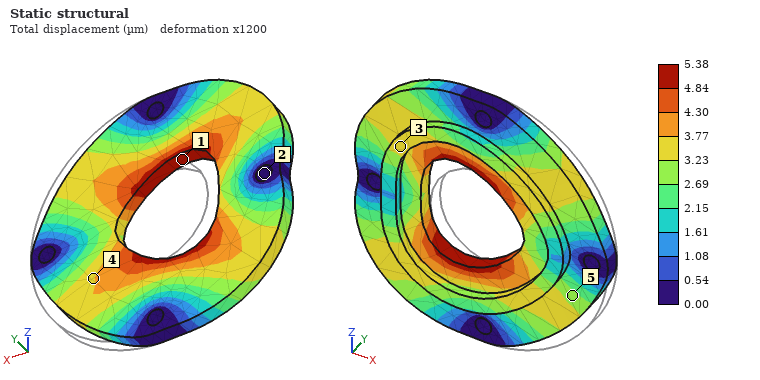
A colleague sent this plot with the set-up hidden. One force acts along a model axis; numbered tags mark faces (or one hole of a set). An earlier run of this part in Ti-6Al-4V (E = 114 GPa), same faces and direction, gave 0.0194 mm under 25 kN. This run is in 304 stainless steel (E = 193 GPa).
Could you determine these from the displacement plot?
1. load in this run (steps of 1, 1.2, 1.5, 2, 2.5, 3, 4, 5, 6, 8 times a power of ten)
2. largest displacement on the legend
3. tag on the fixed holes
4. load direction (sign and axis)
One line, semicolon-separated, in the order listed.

12 kN; 5.38 µm; 2; -X
